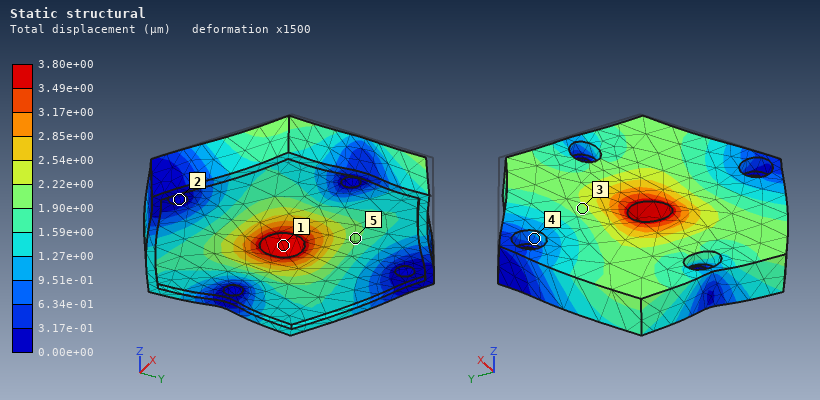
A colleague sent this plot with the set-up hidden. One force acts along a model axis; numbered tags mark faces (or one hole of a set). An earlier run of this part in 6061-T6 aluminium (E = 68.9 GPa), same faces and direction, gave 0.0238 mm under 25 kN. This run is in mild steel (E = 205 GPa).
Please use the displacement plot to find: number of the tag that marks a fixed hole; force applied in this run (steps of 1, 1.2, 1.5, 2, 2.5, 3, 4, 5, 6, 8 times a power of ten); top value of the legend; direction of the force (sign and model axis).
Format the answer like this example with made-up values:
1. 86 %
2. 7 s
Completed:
1. 2
2. 12 kN
3. 3.80e+00 µm
4. -X
